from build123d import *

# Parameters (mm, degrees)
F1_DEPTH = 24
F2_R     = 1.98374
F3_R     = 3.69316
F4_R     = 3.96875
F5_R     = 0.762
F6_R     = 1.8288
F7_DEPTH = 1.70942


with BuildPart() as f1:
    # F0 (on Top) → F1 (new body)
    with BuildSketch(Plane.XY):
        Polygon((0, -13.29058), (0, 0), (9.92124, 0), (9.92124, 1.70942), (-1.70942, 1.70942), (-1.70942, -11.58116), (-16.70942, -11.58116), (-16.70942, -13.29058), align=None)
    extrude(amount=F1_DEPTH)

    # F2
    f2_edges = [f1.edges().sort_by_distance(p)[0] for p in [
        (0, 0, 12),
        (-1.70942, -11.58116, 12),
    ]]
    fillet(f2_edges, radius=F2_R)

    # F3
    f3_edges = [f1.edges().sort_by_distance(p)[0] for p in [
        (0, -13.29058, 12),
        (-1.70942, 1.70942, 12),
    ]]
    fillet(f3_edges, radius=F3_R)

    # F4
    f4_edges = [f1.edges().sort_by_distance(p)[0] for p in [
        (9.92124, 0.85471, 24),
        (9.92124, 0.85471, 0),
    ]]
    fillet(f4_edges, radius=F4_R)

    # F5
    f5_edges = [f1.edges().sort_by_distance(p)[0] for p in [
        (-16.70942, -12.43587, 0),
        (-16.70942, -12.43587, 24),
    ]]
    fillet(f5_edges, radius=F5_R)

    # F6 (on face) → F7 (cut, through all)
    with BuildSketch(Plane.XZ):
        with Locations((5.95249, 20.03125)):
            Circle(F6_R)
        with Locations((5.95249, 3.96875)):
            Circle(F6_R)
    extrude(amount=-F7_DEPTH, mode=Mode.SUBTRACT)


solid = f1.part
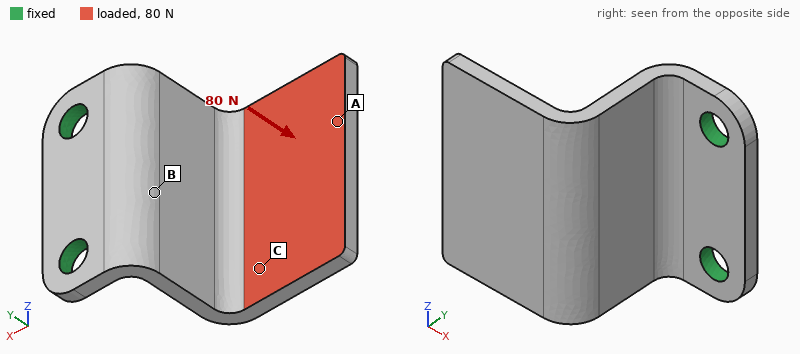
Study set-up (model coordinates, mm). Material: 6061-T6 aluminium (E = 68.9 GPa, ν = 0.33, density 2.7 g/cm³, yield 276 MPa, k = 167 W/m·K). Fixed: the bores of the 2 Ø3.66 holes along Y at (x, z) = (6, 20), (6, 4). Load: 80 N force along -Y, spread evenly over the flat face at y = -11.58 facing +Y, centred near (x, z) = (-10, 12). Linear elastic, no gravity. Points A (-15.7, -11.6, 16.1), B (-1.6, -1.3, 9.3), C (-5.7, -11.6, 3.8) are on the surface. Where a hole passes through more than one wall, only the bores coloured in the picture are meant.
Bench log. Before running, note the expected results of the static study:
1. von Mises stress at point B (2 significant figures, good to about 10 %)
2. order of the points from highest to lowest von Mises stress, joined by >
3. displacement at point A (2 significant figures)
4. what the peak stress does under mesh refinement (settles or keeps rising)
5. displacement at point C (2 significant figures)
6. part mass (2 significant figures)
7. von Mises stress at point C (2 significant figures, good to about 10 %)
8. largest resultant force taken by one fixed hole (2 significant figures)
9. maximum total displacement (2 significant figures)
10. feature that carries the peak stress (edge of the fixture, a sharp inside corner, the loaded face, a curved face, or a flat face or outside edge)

52 MPa
B > C > A
0.40 mm
keeps rising
0.20 mm
4.0 g
29 MPa
40 N
0.44 mm
edge of the fixture
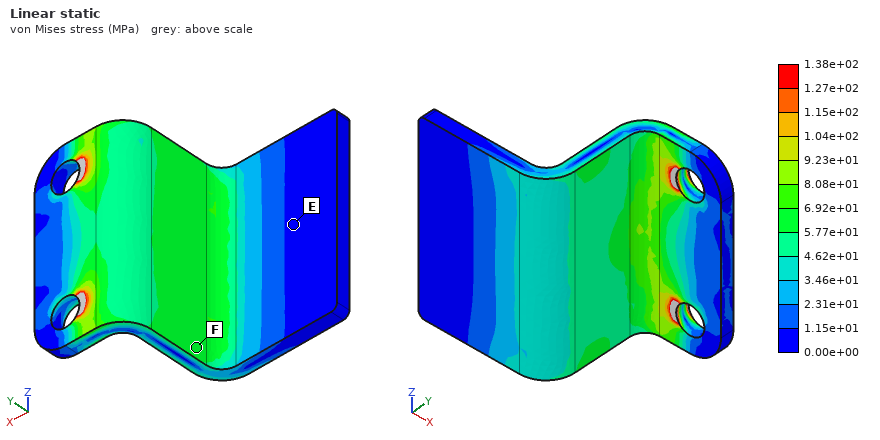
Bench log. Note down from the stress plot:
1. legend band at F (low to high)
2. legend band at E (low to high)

5.77e+01 to 6.92e+01 MPa
0.00e+00 to 1.15e+01 MPa
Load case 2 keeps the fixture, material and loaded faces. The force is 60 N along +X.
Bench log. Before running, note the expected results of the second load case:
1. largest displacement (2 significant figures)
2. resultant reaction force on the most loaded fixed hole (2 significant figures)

0.23 mm
31 N
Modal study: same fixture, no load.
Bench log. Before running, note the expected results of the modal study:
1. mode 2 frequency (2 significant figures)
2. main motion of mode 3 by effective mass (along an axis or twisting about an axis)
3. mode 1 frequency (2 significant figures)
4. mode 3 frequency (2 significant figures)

3900 Hz
along X
1700 Hz
6200 Hz
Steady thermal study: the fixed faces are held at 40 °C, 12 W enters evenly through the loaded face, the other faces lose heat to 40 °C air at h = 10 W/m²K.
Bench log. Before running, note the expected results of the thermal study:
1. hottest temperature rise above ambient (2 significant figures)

46 K
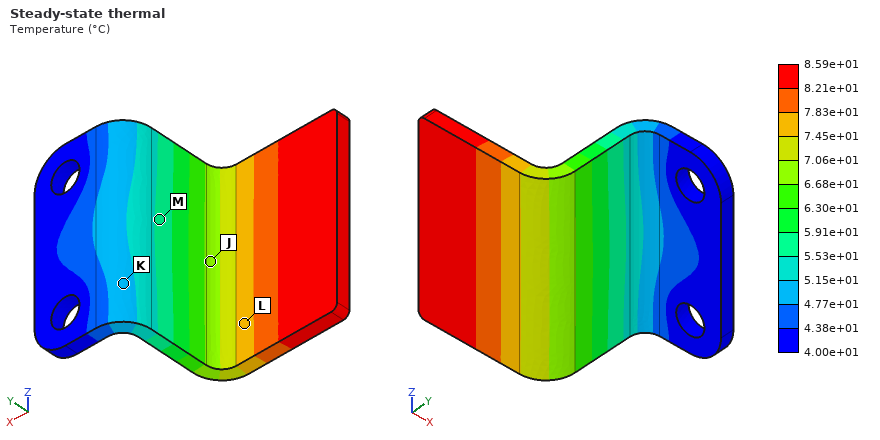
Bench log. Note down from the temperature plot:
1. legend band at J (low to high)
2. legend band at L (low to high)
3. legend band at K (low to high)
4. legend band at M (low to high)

6.68e+01 to 7.06e+01 °C
7.45e+01 to 7.83e+01 °C
4.77e+01 to 5.15e+01 °C
5.53e+01 to 5.91e+01 °C
